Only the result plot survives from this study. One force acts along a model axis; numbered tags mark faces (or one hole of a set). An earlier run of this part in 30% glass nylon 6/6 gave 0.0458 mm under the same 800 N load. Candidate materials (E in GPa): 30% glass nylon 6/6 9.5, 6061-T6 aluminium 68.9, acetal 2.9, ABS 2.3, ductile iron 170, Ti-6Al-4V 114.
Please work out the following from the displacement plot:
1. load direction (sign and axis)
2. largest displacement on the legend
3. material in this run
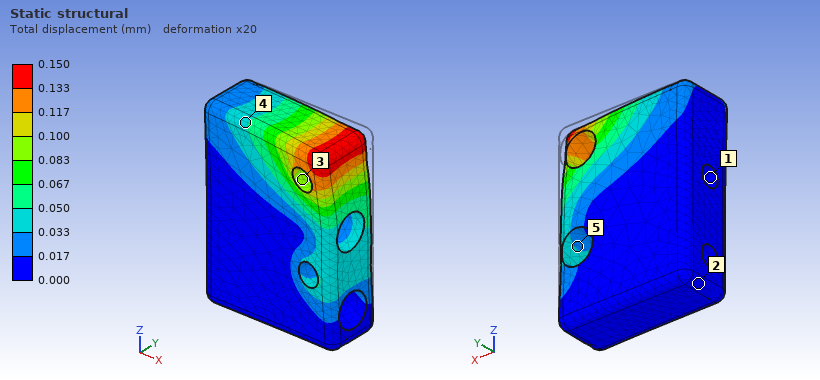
-Y
0.150 mm
acetal
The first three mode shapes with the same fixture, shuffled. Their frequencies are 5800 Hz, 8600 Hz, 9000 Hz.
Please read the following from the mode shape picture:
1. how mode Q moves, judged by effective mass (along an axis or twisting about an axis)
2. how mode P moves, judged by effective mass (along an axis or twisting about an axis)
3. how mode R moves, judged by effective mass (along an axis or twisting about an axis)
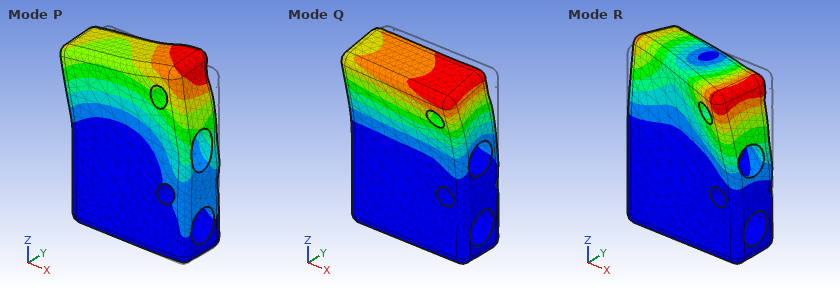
along Y
along X
twisting about Z
